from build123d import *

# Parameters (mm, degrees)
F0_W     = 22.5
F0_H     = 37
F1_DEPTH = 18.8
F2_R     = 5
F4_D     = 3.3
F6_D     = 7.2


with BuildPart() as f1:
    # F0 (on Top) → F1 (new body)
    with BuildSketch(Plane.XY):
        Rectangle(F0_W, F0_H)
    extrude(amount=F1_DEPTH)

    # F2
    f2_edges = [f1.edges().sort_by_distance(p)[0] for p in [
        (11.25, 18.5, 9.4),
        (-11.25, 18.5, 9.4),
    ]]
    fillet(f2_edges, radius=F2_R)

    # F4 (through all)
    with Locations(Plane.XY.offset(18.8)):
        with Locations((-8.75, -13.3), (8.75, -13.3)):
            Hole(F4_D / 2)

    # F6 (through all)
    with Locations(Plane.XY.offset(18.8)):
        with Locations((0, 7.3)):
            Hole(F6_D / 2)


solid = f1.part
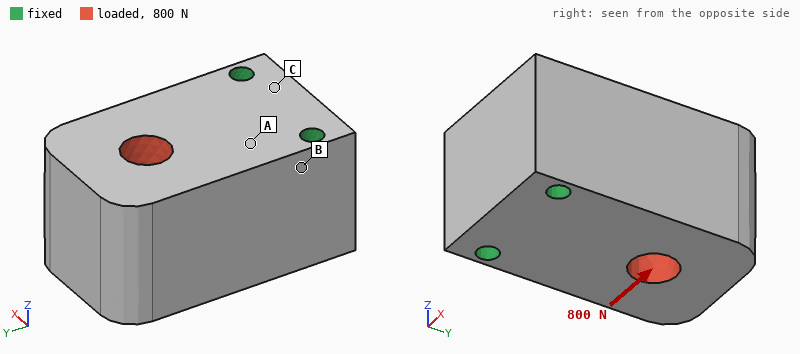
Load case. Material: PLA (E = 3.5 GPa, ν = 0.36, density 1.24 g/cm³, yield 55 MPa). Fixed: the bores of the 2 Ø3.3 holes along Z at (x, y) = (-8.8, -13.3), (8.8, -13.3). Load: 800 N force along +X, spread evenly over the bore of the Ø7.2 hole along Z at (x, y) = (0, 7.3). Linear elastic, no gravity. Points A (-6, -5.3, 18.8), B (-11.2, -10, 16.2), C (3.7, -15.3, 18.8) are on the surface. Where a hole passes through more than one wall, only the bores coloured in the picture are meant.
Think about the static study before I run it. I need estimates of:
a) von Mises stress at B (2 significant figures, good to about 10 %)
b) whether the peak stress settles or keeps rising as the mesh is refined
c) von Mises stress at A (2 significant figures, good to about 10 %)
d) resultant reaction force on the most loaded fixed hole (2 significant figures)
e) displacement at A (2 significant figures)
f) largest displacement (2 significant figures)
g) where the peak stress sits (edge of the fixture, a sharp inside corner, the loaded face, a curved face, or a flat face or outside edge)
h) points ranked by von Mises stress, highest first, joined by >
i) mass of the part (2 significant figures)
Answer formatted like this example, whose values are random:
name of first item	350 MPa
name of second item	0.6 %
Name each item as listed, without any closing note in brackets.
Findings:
von Mises stress at B	7.8 MPa
whether the peak stress settles or keeps rising as the mesh is refined	keeps rising
von Mises stress at A	4.4 MPa
resultant reaction force on the most loaded fixed hole	970 N
displacement at A	0.018 mm
largest displacement	0.10 mm
where the peak stress sits	edge of the fixture
points ranked by von Mises stress, highest first, joined by >	B > A > C
mass of the part	18 g
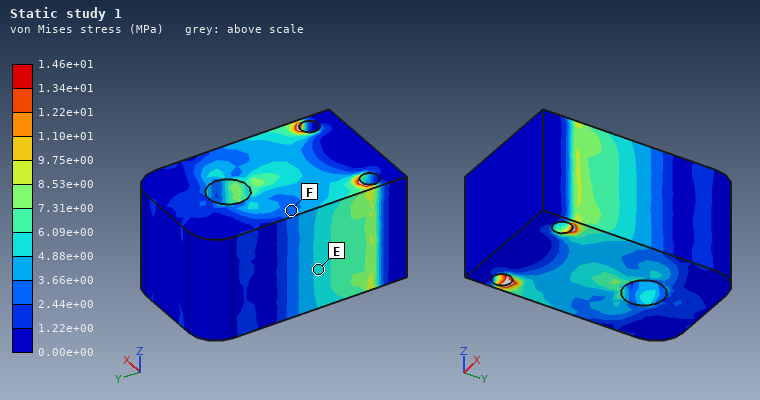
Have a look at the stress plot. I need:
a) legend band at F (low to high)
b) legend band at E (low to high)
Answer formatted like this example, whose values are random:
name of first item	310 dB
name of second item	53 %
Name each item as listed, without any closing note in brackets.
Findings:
legend band at F	2.44e+00 to 3.66e+00 MPa
legend band at E	4.88e+00 to 6.09e+00 MPa
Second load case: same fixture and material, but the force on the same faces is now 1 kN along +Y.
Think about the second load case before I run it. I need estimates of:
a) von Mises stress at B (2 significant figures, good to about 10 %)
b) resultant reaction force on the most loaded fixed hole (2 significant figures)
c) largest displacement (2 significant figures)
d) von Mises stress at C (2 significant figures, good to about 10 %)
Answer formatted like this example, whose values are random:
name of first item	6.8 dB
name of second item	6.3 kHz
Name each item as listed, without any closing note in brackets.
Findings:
von Mises stress at B	2.6 MPa
resultant reaction force on the most loaded fixed hole	510 N
largest displacement	24 µm
von Mises stress at C	1.3 MPa
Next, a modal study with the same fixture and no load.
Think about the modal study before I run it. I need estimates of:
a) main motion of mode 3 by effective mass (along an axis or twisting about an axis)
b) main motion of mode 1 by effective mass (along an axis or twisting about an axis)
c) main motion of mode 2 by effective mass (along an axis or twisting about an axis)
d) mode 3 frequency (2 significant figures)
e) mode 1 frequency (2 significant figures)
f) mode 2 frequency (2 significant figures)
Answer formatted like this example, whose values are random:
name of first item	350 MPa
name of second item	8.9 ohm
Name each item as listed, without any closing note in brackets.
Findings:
main motion of mode 3 by effective mass	twisting about Y
main motion of mode 1 by effective mass	along Z
main motion of mode 2 by effective mass	along X
mode 3 frequency	7500 Hz
mode 1 frequency	4000 Hz
mode 2 frequency	4900 Hz
